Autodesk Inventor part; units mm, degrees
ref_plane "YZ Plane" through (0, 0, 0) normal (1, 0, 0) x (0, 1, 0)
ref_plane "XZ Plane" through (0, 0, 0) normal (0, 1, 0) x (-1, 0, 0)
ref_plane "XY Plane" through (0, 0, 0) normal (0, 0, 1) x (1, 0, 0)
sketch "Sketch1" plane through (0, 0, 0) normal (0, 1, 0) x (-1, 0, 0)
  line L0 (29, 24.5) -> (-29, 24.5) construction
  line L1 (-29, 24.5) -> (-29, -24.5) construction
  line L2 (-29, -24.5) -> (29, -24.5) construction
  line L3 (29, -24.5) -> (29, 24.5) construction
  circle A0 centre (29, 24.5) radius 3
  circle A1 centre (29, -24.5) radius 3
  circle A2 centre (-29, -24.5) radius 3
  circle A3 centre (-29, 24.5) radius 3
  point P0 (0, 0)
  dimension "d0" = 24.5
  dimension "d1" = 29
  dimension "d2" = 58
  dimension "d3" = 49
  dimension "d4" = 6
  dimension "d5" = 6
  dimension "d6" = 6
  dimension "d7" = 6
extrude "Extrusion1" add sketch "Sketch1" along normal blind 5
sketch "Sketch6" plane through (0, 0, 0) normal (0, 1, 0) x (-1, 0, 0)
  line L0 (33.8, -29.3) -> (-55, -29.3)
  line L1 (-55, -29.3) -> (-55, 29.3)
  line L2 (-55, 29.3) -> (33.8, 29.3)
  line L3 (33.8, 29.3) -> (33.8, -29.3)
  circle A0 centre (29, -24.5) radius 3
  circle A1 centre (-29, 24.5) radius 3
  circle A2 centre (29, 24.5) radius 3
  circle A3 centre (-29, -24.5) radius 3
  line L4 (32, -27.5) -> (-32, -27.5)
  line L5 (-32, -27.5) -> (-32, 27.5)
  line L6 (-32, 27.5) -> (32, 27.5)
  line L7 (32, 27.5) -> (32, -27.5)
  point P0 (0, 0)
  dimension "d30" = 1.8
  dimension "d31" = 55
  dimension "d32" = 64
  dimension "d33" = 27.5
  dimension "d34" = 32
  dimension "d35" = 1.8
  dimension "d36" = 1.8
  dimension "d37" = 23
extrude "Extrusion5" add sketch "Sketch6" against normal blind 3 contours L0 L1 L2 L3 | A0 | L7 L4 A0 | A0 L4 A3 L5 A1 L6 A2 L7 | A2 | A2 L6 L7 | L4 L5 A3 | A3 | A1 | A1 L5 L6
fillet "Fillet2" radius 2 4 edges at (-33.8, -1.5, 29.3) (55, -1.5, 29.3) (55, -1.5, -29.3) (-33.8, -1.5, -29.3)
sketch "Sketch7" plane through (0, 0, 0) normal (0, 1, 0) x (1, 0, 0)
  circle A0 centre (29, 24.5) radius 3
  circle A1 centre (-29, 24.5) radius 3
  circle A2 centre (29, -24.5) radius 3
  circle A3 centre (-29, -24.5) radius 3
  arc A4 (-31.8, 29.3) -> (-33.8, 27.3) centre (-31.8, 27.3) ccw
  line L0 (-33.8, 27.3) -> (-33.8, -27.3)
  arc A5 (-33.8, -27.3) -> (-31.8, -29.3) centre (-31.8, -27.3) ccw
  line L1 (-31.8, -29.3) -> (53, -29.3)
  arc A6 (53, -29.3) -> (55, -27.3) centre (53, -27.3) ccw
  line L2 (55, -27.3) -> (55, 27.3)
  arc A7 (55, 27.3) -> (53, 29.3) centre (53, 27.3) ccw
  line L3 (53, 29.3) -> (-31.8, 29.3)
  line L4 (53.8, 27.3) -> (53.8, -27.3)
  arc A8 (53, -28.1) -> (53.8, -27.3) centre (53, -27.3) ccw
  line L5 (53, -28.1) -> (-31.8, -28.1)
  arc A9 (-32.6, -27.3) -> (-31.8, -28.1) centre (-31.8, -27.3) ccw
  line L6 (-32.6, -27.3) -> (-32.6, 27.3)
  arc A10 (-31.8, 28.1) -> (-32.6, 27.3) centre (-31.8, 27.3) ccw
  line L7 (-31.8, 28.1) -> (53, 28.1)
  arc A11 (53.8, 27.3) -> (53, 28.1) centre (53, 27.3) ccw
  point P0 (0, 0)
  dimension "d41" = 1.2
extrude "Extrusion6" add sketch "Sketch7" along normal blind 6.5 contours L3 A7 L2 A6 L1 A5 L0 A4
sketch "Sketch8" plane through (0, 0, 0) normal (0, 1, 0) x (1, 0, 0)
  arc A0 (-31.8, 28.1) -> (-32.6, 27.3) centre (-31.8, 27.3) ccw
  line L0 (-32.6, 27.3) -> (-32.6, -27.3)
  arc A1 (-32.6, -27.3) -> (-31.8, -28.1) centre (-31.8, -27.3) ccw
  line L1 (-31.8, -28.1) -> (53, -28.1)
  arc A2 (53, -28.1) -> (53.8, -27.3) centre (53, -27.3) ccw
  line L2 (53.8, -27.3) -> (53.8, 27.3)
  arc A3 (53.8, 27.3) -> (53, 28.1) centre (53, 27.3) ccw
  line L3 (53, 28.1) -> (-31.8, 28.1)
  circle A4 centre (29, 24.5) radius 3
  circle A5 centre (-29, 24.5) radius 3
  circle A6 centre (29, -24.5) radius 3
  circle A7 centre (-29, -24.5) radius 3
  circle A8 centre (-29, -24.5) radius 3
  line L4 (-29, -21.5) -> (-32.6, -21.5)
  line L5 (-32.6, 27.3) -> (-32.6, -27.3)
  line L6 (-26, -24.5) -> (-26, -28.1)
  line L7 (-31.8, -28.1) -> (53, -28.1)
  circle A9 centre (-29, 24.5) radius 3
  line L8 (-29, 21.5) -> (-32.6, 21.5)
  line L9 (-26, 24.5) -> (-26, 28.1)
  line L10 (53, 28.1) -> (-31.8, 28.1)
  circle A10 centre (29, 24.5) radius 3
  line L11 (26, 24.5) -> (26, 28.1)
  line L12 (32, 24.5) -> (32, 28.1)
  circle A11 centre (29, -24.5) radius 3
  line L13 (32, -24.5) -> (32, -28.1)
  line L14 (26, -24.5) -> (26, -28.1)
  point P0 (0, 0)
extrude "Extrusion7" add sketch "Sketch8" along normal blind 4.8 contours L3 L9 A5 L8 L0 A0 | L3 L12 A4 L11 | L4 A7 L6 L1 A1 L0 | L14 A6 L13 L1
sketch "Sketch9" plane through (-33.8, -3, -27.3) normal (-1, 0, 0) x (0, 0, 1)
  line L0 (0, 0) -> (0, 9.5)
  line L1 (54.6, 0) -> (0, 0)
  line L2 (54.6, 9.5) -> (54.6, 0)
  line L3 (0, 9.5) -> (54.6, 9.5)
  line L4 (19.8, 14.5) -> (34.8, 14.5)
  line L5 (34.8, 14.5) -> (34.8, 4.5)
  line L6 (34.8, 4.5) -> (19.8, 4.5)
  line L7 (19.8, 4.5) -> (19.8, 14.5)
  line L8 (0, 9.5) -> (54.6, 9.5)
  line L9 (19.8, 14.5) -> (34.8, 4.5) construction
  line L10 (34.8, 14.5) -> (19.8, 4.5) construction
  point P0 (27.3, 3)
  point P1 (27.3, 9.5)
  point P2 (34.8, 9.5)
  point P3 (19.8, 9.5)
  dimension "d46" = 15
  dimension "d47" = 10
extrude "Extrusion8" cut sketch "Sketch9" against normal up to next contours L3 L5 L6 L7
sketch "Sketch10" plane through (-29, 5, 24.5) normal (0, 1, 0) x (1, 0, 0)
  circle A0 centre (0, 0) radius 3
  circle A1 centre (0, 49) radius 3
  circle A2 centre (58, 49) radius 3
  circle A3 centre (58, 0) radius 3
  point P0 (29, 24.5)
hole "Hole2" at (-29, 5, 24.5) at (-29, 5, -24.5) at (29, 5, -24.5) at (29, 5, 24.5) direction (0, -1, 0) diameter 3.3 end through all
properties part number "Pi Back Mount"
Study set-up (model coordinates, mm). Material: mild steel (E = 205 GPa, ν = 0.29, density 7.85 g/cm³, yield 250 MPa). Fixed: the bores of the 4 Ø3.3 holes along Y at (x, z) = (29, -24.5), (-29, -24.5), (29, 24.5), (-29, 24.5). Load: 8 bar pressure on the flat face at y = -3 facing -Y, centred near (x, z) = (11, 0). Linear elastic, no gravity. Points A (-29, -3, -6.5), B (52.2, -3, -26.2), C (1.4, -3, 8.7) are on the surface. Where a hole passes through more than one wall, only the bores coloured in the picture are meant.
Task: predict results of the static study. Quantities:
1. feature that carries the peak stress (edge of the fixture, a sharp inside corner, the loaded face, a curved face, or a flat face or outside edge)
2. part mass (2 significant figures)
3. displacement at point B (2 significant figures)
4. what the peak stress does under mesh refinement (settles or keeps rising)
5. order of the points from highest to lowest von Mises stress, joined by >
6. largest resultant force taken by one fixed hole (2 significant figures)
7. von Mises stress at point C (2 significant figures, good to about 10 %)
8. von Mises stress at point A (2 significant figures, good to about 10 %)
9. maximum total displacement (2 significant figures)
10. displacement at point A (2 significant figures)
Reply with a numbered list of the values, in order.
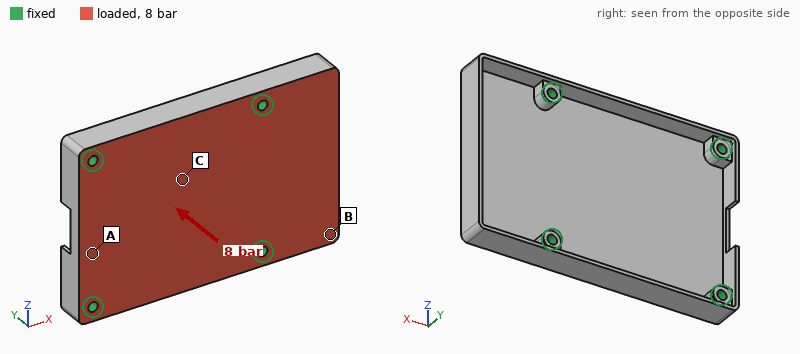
1. edge of the fixture
2. 140 g
3. 31 µm
4. keeps rising
5. C > A > B
6. 1.4 kN
7. 67 MPa
8. 35 MPa
9. 71 µm
10. 19 µm
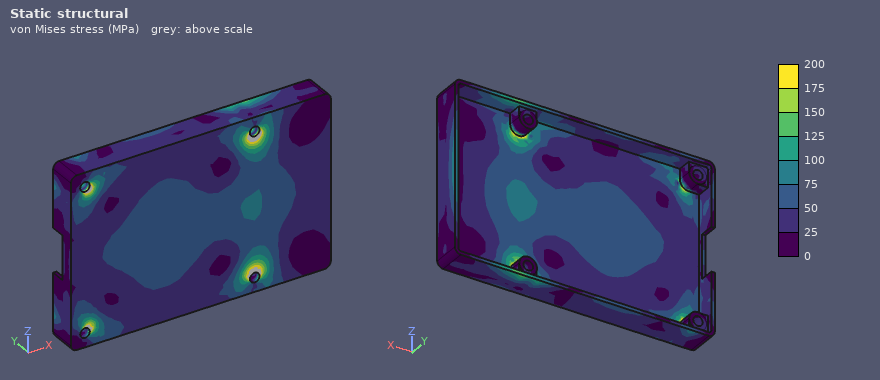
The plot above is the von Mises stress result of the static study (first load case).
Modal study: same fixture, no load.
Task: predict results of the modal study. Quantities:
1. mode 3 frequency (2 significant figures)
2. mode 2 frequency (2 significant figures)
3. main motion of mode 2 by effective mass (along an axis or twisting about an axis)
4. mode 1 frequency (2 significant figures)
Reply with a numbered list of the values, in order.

1. 7100 Hz
2. 4300 Hz
3. along Y
4. 3900 Hz
